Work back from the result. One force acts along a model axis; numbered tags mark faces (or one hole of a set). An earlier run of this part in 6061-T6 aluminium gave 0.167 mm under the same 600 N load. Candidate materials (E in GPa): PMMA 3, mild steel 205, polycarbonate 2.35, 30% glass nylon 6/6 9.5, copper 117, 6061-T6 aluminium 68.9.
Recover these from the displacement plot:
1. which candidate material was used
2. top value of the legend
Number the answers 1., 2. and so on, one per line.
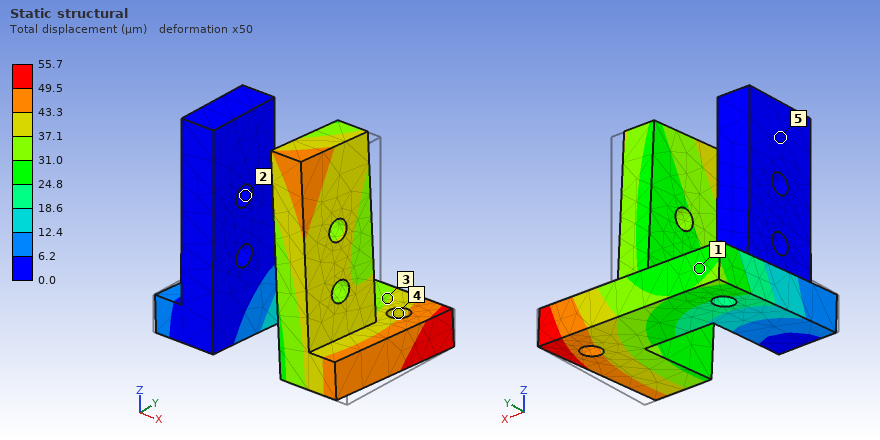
1. mild steel
2. 55.7 µm
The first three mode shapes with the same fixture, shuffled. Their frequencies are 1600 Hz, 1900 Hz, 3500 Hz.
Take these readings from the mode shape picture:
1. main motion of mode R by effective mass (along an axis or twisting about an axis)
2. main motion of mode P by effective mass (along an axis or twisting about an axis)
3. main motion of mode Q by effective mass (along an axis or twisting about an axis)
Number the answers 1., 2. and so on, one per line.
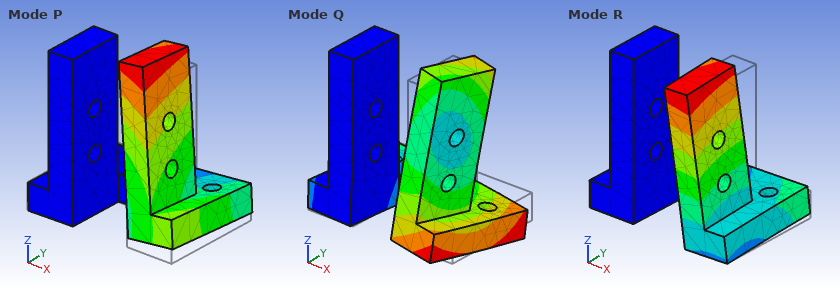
1. along Y
2. along Z
3. along Y
